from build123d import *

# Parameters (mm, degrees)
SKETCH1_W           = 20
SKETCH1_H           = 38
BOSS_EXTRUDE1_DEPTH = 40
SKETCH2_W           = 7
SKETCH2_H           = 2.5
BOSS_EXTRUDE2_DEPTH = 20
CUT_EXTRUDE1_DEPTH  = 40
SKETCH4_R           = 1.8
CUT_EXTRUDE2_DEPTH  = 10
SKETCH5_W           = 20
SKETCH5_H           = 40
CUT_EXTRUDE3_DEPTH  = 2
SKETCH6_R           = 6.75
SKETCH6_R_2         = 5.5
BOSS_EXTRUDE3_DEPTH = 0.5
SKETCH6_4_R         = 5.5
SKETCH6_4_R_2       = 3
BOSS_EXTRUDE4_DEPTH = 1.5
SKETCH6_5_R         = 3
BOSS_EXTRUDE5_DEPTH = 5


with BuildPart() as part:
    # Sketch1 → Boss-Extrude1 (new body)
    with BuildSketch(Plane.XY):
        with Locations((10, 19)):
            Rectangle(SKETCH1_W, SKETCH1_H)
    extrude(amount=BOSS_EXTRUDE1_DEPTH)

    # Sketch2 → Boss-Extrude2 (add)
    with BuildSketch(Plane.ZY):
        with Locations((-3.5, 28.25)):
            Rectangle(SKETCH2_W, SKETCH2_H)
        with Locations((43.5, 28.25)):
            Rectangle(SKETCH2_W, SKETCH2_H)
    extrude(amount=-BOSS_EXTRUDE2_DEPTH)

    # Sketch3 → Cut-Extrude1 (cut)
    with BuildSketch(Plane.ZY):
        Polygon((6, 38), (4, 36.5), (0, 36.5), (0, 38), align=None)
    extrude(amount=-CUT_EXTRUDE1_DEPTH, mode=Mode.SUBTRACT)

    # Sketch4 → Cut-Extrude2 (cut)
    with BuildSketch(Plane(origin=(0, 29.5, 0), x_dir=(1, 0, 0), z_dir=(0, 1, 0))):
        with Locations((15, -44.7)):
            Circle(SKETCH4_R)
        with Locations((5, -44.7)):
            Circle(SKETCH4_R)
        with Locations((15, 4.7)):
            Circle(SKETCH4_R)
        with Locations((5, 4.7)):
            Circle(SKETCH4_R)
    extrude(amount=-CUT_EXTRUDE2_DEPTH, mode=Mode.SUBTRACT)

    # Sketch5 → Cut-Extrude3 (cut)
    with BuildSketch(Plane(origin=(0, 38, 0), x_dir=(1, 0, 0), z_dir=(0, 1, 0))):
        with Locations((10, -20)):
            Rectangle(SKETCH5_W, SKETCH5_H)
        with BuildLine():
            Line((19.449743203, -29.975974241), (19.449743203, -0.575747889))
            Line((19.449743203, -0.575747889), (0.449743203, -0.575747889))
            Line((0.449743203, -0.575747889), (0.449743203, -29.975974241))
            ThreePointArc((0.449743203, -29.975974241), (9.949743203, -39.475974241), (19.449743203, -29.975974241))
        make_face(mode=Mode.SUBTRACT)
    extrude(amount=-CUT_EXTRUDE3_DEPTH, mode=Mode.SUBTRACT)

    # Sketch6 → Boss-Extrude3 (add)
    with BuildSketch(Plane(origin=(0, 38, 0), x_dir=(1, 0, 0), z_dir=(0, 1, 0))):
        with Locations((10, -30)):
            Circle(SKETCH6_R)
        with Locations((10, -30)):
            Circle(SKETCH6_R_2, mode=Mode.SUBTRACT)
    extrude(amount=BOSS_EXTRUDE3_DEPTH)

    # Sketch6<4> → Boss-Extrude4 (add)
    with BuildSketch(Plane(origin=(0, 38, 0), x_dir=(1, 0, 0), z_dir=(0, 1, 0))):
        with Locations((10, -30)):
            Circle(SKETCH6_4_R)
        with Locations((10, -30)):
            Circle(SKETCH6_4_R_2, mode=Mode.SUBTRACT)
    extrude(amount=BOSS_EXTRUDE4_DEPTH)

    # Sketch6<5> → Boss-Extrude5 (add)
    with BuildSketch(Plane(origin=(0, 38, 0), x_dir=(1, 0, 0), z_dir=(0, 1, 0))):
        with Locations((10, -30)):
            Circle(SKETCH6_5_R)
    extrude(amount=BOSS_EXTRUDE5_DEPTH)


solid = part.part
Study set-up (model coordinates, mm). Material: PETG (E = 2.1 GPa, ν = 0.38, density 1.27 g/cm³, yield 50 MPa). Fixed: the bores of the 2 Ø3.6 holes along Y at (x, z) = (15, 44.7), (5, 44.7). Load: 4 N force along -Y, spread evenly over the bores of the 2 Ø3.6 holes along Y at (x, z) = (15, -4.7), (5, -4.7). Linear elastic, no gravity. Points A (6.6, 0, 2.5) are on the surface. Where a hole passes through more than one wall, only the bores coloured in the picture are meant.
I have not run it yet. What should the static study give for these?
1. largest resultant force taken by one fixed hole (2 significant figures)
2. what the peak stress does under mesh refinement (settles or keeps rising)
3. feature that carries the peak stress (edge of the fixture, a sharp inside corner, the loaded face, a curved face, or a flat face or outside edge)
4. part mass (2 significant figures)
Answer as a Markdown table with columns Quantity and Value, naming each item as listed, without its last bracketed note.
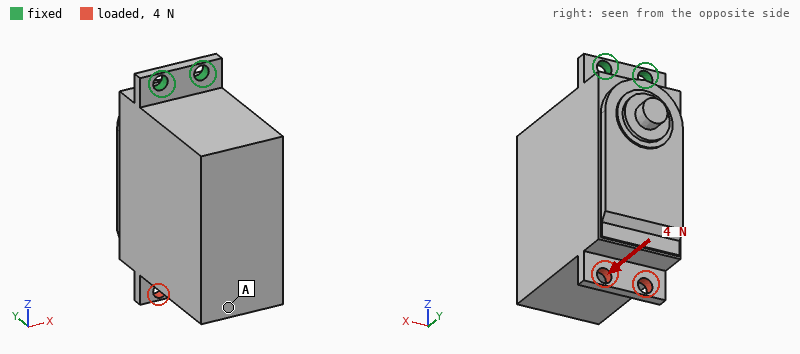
| Quantity | Value |
|---|---|
| largest resultant force taken by one fixed hole | 2.0 N |
| what the peak stress does under mesh refinement | keeps rising |
| feature that carries the peak stress | edge of the fixture |
| part mass | 39 g |
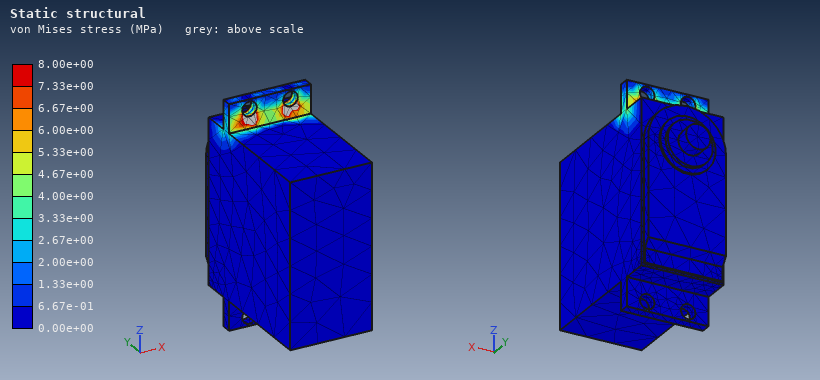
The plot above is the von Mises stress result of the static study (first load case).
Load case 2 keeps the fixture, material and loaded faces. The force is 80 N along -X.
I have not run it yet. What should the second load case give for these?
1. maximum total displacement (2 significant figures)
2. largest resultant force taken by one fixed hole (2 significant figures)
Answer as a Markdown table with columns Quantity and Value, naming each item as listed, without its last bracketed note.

| Quantity | Value |
|---|---|
| maximum total displacement | 0.57 mm |
| largest resultant force taken by one fixed hole | 320 N |
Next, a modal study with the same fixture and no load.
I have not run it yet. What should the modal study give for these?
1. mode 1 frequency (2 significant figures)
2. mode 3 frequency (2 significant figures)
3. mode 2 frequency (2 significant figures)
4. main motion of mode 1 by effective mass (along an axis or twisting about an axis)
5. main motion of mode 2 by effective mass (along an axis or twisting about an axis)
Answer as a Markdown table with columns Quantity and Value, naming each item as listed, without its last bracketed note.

| Quantity | Value |
|---|---|
| mode 1 frequency | 100 Hz |
| mode 3 frequency | 820 Hz |
| mode 2 frequency | 460 Hz |
| main motion of mode 1 by effective mass | along Y |
| main motion of mode 2 by effective mass | along X |
